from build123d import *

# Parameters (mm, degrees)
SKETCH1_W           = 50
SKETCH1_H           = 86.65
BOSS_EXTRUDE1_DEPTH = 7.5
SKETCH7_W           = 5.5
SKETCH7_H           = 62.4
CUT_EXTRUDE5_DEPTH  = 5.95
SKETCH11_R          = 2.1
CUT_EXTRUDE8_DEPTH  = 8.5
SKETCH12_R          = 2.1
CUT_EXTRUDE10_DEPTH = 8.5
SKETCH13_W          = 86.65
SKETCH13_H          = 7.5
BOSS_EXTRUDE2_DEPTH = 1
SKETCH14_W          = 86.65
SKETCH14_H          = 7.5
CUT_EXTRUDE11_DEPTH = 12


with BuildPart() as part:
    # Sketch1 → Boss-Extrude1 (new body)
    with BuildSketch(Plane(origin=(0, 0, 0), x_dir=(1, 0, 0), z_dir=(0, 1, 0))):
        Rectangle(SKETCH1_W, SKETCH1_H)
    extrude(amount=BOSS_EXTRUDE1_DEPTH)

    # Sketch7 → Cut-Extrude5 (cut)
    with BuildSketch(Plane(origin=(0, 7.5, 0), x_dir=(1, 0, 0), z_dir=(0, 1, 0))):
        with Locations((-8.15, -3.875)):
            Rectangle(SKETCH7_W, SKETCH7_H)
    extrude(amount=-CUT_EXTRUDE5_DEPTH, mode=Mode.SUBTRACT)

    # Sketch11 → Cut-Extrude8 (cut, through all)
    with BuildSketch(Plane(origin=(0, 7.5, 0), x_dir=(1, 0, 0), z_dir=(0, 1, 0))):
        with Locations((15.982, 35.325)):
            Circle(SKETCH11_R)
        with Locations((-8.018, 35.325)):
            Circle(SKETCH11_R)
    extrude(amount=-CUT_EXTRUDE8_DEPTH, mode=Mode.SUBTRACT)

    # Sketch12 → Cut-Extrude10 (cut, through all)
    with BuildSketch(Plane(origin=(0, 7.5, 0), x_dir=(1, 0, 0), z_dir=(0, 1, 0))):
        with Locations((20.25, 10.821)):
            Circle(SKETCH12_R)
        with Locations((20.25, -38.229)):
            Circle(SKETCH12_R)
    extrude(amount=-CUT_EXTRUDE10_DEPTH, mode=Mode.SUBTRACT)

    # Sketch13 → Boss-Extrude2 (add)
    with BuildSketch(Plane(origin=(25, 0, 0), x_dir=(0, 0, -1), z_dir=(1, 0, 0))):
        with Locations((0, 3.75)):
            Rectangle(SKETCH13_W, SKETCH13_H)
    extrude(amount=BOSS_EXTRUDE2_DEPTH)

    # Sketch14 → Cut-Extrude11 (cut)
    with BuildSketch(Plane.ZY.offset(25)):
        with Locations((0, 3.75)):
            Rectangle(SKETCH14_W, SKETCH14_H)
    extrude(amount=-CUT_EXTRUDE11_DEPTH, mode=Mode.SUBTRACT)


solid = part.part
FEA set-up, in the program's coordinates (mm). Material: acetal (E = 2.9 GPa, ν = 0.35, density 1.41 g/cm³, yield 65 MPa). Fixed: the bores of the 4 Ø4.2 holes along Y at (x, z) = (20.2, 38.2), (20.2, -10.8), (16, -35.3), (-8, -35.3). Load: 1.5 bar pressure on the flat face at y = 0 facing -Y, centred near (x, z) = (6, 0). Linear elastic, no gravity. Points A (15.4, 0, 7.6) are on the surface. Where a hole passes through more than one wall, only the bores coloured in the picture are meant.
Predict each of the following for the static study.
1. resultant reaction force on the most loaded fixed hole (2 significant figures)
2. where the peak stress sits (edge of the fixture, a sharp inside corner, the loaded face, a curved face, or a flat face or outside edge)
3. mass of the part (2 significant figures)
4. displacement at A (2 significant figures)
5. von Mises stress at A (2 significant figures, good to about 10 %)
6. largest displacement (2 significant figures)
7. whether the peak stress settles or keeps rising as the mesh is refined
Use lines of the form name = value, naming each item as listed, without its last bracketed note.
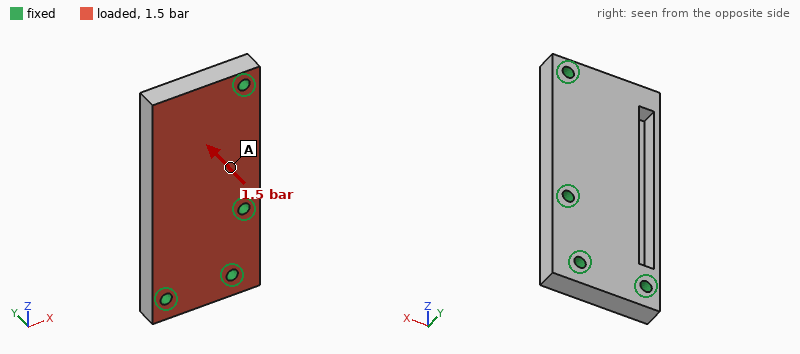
resultant reaction force on the most loaded fixed hole = 180 N
where the peak stress sits = edge of the fixture
mass of the part = 32 g
displacement at A = 0.070 mm
von Mises stress at A = 2.6 MPa
largest displacement = 0.38 mm
whether the peak stress settles or keeps rising as the mesh is refined = keeps rising
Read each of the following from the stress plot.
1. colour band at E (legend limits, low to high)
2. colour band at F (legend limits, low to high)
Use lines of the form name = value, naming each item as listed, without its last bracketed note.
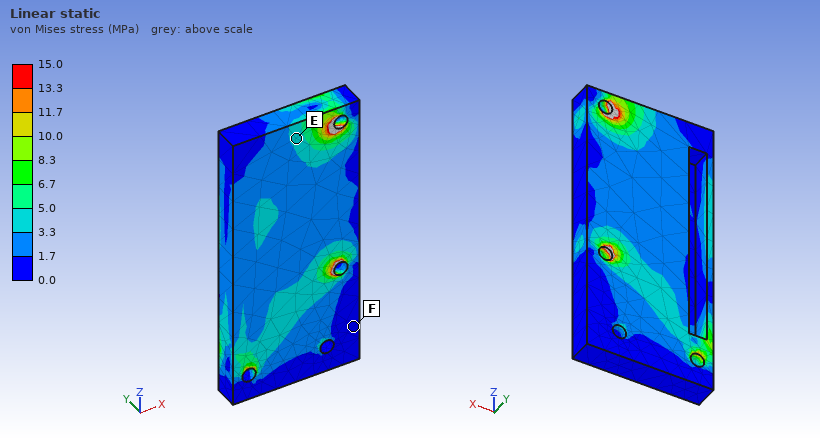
colour band at E = 3.3 to 5.0 MPa
colour band at F = 0.0 to 1.7 MPa
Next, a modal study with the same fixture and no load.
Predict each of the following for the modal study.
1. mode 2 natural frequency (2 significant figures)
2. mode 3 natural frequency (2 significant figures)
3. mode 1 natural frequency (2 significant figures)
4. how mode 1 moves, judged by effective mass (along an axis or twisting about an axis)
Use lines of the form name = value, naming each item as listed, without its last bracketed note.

mode 2 natural frequency = 2900 Hz
mode 3 natural frequency = 3500 Hz
mode 1 natural frequency = 1500 Hz
how mode 1 moves, judged by effective mass = along Y
